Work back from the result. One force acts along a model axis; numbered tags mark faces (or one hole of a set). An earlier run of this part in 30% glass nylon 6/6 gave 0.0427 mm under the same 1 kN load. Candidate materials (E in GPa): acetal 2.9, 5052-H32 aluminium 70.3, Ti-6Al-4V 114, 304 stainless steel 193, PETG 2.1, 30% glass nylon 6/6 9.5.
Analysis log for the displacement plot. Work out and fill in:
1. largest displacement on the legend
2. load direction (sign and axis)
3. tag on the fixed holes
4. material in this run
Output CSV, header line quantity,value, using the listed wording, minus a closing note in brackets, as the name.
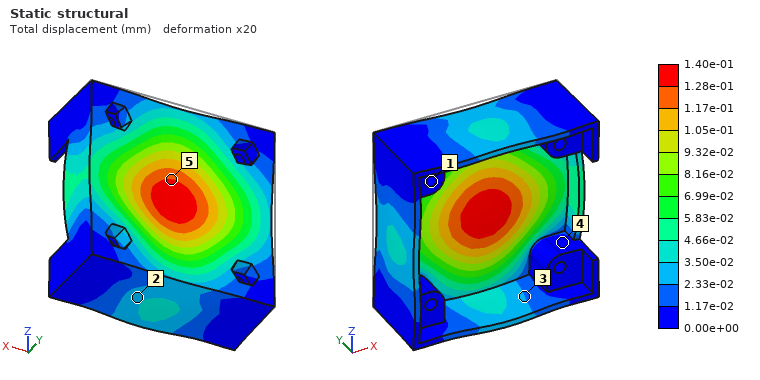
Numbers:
quantity,value
largest displacement on the legend,1.40e-01 mm
load direction,-Y
tag on the fixed holes,1
material in this run,acetal
